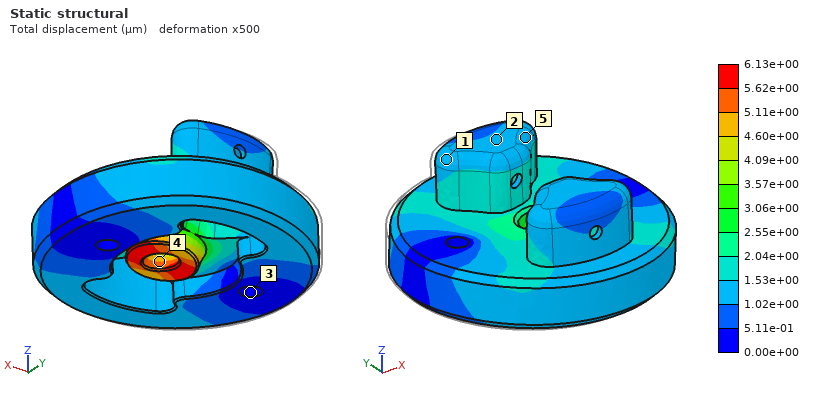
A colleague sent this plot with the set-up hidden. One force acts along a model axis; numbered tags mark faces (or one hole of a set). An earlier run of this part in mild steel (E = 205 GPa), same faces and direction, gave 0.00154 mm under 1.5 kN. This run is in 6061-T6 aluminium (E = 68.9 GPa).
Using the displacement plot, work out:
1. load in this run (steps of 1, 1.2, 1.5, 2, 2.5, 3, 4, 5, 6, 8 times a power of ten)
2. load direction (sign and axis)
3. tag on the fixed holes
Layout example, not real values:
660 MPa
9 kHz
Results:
2 kN
+X
3
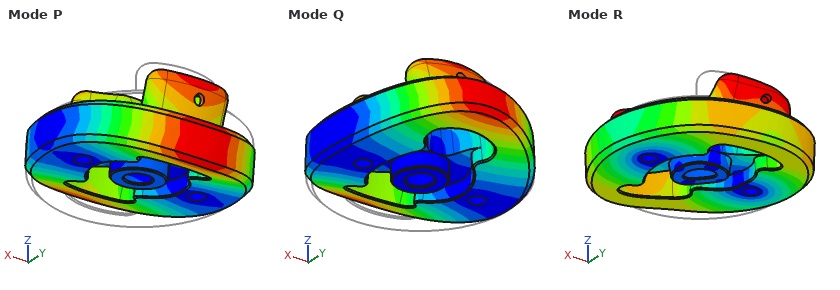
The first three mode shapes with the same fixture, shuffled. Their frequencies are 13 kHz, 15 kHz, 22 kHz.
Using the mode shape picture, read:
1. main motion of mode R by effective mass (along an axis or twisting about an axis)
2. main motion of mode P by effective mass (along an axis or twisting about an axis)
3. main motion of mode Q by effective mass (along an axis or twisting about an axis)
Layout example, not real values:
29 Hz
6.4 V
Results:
twisting about Z
twisting about X
along Z
